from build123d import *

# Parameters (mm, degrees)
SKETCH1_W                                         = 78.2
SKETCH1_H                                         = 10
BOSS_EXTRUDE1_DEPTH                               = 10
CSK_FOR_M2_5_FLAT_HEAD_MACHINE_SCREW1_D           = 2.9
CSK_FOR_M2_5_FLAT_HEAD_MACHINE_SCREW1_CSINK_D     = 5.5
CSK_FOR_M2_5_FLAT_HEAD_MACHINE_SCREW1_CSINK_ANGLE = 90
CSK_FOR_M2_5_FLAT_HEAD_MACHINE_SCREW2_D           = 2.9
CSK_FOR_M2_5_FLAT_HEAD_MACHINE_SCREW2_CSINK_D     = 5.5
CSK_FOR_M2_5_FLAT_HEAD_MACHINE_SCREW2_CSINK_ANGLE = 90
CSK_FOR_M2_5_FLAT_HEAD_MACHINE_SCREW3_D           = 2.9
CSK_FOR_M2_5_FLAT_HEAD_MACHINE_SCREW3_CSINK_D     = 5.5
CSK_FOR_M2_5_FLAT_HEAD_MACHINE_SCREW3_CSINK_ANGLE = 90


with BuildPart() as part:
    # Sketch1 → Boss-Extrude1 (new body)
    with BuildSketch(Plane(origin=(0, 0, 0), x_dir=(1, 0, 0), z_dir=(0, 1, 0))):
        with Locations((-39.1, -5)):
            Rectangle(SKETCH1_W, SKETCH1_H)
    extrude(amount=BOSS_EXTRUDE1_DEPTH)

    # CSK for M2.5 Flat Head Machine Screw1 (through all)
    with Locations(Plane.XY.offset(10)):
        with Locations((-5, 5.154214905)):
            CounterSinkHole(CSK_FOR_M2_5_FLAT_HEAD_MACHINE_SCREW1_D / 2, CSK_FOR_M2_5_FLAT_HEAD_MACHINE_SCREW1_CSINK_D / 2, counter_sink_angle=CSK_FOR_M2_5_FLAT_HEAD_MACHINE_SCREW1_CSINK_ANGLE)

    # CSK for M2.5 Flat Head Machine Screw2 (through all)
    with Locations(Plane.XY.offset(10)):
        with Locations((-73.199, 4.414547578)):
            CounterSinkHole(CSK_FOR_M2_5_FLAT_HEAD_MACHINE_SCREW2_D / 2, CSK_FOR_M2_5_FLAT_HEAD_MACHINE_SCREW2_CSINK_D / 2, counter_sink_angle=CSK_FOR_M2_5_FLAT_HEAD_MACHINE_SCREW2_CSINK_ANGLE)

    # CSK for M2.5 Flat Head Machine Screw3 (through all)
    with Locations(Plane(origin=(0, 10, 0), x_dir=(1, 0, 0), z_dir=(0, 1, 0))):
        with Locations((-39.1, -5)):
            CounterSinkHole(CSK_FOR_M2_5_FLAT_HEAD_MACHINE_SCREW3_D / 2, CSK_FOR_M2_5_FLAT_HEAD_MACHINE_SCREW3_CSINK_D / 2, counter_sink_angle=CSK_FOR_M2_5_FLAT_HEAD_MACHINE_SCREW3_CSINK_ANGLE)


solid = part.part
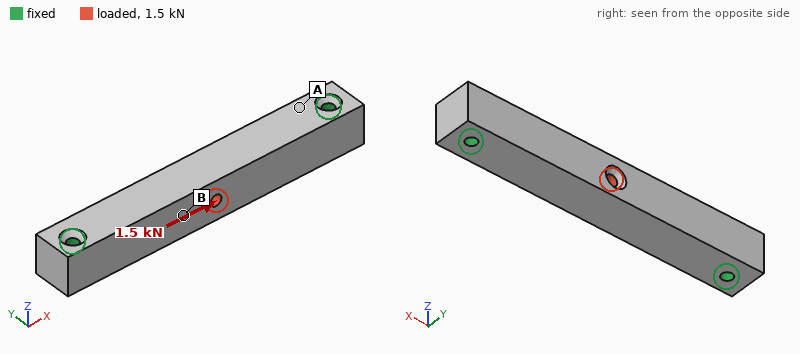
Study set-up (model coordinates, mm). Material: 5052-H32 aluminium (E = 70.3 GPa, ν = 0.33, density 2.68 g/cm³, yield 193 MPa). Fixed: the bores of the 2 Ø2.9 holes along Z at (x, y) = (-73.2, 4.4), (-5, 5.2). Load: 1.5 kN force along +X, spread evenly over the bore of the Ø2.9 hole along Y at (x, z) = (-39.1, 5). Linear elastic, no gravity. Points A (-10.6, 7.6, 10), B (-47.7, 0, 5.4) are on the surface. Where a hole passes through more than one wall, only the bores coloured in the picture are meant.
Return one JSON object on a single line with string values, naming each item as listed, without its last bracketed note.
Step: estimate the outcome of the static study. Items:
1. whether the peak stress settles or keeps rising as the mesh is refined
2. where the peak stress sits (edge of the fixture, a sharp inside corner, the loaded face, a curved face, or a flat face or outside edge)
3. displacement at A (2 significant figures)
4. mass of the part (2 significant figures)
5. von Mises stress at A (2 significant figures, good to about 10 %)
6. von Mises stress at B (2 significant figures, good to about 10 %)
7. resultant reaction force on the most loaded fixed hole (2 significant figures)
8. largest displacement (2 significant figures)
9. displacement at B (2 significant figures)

{"whether the peak stress settles or keeps rising as the mesh is refined": "keeps rising", "where the peak stress sits": "edge of the fixture", "displacement at A": "0.87 µm", "mass of the part": "20 g", "von Mises stress at A": "6.5 MPa", "von Mises stress at B": "11 MPa", "resultant reaction force on the most loaded fixed hole": "750 N", "largest displacement": "4.6 µm", "displacement at B": "3.2 µm"}
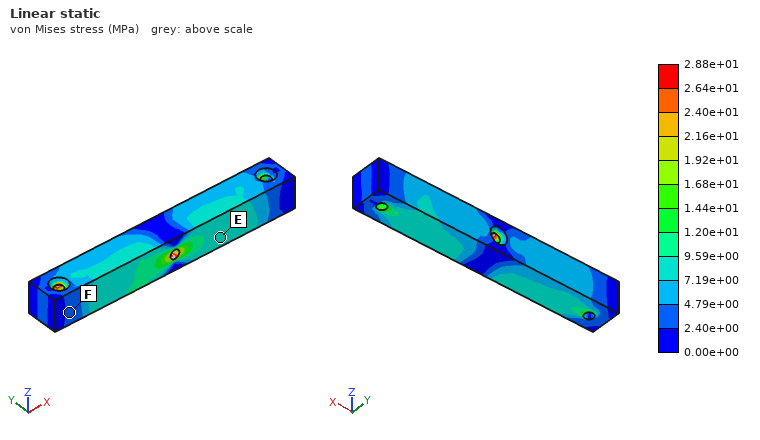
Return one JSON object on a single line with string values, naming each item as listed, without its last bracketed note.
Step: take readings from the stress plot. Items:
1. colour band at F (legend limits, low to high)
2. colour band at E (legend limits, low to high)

{"colour band at F": "2.40e+00 to 4.79e+00 MPa", "colour band at E": "7.19e+00 to 9.59e+00 MPa"}
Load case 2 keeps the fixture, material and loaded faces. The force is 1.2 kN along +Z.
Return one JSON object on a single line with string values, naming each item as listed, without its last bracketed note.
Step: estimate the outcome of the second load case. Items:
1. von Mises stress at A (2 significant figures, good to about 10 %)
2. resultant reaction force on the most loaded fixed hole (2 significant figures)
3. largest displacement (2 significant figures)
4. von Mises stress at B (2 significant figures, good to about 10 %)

{"von Mises stress at A": "35 MPa", "resultant reaction force on the most loaded fixed hole": "600 N", "largest displacement": "49 µm", "von Mises stress at B": "21 MPa"}
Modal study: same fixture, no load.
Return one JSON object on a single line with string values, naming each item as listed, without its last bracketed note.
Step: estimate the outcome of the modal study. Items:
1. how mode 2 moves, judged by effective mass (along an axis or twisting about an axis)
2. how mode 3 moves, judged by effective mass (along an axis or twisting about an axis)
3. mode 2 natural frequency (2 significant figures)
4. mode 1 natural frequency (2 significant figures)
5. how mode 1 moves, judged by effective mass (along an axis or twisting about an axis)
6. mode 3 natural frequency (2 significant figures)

{"how mode 2 moves, judged by effective mass": "along Z", "how mode 3 moves, judged by effective mass": "twisting about X", "mode 2 natural frequency": "9600 Hz", "mode 1 natural frequency": "7900 Hz", "how mode 1 moves, judged by effective mass": "along Y", "mode 3 natural frequency": "21 kHz"}
